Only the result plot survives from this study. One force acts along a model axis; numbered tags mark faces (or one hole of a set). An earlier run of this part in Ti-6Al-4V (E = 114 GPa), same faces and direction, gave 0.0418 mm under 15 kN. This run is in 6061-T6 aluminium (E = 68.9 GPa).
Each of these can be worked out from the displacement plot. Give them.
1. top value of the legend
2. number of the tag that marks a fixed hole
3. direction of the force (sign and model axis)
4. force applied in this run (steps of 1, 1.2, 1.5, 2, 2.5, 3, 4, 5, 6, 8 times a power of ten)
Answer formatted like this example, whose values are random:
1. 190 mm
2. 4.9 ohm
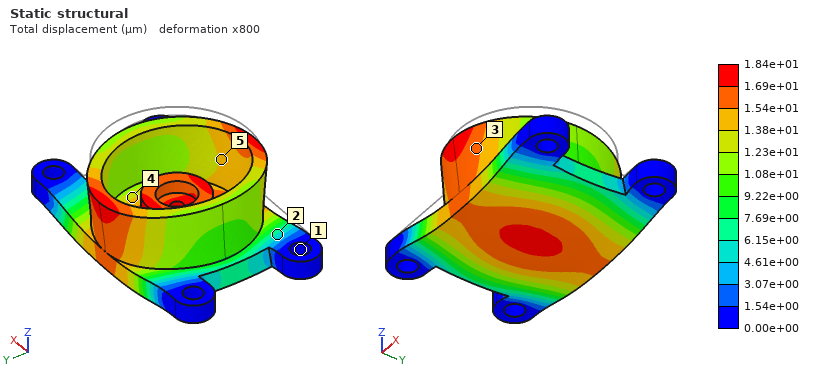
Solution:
1. 1.84e+01 µm
2. 1
3. -Z
4. 4 kN
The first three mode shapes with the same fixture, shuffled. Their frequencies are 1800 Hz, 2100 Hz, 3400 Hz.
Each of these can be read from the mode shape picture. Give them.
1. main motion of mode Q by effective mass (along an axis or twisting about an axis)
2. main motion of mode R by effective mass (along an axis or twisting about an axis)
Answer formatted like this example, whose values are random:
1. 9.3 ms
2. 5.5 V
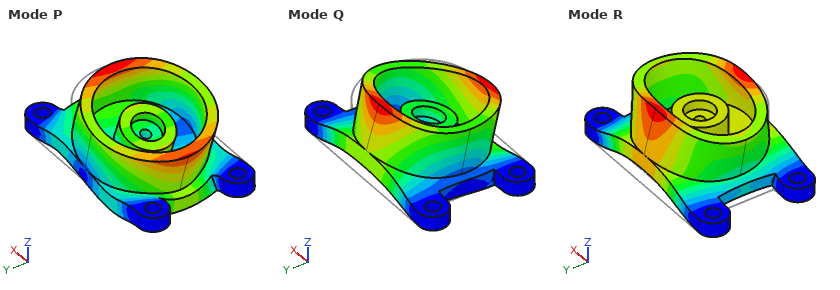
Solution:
1. along Y
2. along Z
